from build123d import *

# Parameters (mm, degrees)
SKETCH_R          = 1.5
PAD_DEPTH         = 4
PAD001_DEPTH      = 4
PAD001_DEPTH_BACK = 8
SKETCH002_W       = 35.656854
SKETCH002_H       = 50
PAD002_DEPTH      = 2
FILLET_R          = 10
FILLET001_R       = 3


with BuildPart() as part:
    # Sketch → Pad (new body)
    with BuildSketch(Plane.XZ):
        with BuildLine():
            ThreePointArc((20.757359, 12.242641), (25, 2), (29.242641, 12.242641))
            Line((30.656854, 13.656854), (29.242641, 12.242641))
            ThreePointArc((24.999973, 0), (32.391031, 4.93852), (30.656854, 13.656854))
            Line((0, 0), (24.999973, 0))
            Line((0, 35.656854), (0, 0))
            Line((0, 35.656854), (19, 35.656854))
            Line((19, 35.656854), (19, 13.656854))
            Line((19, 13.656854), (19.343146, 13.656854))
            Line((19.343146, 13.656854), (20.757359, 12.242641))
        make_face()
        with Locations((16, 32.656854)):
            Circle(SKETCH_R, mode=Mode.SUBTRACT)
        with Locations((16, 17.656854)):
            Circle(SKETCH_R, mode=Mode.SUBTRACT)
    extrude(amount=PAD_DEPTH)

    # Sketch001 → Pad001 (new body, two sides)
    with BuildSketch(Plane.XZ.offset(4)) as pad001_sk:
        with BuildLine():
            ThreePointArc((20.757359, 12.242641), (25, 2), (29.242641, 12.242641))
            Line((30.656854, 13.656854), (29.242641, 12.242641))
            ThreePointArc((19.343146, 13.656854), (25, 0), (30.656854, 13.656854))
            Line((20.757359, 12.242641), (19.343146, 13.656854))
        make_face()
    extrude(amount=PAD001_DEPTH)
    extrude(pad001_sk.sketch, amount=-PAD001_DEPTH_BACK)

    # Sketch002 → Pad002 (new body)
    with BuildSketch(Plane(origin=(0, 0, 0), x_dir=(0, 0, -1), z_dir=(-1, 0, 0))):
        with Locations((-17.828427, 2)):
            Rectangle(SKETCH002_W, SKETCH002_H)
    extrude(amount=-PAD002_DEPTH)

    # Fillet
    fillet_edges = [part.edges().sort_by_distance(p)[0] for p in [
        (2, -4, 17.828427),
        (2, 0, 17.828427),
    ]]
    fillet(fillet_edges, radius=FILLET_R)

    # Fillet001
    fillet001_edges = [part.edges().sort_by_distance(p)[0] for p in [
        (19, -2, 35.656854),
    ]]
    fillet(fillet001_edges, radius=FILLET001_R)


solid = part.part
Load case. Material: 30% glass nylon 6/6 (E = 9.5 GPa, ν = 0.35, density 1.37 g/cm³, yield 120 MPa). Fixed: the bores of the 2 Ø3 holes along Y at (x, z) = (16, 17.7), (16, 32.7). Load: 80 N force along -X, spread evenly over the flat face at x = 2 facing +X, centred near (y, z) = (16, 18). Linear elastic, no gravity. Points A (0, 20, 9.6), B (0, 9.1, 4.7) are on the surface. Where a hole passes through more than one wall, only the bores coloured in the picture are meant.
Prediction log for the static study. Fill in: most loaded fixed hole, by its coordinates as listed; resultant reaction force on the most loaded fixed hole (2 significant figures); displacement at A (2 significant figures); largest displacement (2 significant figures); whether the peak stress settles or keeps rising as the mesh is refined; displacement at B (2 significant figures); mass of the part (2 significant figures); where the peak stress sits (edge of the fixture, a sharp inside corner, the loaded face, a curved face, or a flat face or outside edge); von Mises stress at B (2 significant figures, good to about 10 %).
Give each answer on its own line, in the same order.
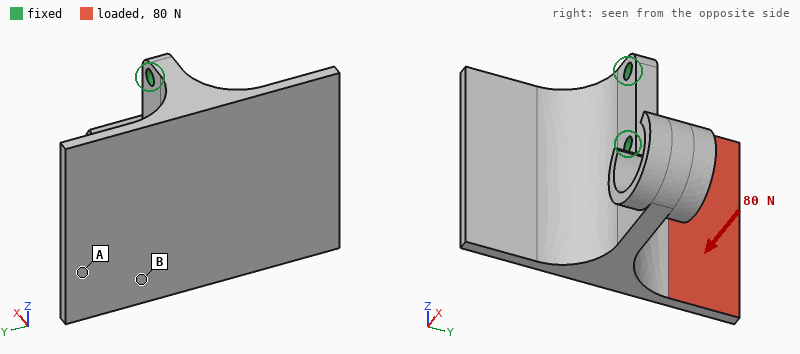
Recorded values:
(16, 17.7)
75 N
0.42 mm
0.51 mm
keeps rising
0.18 mm
11 g
edge of the fixture
20 MPa
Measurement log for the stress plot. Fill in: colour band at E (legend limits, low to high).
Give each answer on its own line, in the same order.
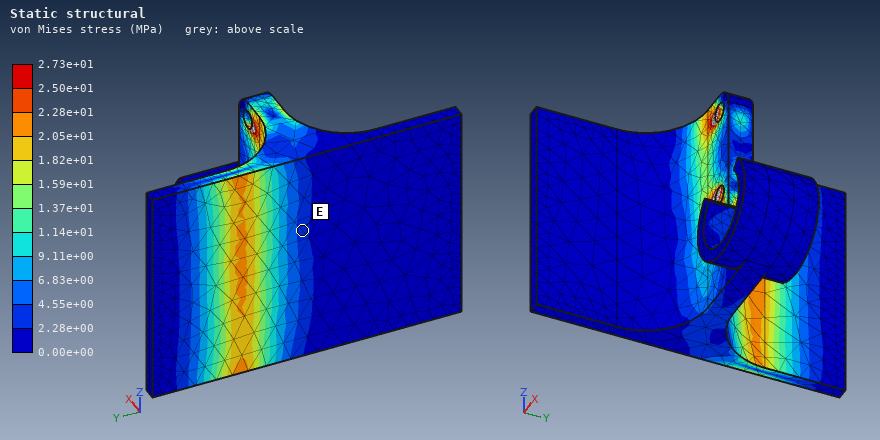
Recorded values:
2.28e+00 to 4.55e+00 MPa
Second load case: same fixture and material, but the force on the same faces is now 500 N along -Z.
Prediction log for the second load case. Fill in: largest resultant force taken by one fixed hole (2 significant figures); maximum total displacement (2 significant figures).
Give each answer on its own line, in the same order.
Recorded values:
690 N
0.71 mm
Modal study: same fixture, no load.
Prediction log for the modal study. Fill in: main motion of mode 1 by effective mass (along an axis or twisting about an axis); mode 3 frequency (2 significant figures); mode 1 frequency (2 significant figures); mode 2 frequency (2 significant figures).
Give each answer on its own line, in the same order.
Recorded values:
along Y
2400 Hz
1400 Hz
2300 Hz
